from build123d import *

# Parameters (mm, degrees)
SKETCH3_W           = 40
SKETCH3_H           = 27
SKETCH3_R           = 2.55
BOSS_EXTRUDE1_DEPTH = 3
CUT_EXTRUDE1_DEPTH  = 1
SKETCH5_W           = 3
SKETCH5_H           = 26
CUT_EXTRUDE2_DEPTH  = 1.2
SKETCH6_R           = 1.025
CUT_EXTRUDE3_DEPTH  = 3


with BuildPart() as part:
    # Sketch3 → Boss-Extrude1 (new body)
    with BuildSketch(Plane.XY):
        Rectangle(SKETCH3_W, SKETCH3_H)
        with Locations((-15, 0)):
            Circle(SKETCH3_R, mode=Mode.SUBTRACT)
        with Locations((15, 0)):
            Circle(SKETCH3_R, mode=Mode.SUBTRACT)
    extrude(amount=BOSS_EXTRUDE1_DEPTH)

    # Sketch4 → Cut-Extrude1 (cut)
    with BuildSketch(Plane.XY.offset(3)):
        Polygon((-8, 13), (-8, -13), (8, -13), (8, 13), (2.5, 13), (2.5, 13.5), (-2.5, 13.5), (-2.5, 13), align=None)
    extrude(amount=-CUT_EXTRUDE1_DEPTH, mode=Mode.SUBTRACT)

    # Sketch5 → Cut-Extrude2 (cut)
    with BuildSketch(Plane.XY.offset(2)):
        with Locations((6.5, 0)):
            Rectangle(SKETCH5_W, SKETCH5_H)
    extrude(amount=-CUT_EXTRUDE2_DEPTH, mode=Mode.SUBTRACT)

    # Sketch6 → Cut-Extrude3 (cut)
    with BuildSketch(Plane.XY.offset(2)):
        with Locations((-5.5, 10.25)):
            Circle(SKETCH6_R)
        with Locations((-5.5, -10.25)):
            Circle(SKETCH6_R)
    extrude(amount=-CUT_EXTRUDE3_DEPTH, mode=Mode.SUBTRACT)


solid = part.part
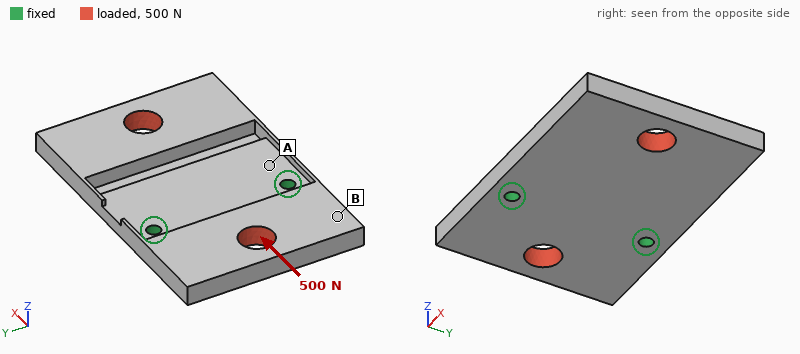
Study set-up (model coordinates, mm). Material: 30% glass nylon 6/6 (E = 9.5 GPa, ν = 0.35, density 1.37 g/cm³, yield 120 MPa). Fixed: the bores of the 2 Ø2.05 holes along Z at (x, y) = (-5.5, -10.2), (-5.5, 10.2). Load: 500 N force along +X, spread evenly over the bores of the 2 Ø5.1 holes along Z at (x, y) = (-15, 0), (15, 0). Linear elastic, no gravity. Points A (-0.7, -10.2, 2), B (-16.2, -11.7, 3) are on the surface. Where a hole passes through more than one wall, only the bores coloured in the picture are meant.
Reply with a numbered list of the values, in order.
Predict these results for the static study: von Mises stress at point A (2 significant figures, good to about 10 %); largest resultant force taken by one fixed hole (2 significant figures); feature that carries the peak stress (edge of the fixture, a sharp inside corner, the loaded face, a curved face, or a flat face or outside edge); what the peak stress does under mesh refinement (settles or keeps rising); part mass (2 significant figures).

1. 16 MPa
2. 250 N
3. a sharp inside corner
4. keeps rising
5. 3.6 g
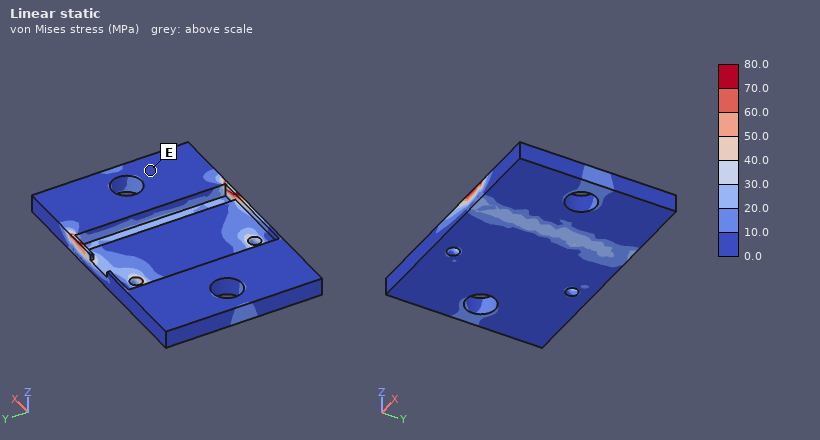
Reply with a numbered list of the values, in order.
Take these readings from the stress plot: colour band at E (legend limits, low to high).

1. 0.0 to 10.0 MPa
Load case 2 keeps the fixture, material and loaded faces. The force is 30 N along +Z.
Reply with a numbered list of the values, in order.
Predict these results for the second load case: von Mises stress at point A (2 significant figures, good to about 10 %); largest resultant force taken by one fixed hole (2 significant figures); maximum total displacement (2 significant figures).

1. 12 MPa
2. 16 N
3. 0.47 mm
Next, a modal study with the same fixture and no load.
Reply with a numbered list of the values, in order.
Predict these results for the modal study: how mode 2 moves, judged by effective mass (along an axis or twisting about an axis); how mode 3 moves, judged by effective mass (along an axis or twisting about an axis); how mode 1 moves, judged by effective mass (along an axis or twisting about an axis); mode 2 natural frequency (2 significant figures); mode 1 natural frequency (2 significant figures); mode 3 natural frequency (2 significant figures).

1. twisting about X
2. along Z
3. along Z
4. 2900 Hz
5. 970 Hz
6. 3500 Hz
